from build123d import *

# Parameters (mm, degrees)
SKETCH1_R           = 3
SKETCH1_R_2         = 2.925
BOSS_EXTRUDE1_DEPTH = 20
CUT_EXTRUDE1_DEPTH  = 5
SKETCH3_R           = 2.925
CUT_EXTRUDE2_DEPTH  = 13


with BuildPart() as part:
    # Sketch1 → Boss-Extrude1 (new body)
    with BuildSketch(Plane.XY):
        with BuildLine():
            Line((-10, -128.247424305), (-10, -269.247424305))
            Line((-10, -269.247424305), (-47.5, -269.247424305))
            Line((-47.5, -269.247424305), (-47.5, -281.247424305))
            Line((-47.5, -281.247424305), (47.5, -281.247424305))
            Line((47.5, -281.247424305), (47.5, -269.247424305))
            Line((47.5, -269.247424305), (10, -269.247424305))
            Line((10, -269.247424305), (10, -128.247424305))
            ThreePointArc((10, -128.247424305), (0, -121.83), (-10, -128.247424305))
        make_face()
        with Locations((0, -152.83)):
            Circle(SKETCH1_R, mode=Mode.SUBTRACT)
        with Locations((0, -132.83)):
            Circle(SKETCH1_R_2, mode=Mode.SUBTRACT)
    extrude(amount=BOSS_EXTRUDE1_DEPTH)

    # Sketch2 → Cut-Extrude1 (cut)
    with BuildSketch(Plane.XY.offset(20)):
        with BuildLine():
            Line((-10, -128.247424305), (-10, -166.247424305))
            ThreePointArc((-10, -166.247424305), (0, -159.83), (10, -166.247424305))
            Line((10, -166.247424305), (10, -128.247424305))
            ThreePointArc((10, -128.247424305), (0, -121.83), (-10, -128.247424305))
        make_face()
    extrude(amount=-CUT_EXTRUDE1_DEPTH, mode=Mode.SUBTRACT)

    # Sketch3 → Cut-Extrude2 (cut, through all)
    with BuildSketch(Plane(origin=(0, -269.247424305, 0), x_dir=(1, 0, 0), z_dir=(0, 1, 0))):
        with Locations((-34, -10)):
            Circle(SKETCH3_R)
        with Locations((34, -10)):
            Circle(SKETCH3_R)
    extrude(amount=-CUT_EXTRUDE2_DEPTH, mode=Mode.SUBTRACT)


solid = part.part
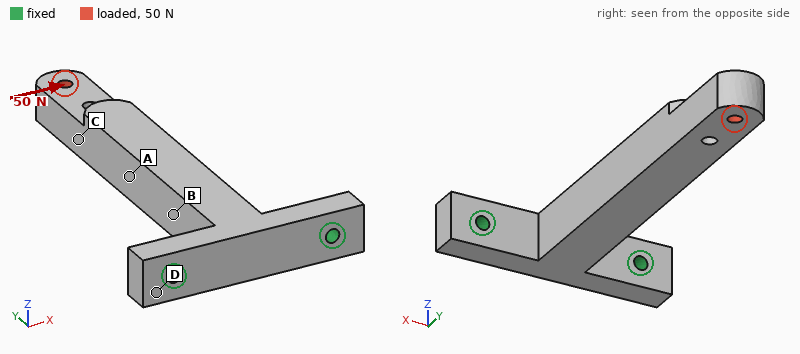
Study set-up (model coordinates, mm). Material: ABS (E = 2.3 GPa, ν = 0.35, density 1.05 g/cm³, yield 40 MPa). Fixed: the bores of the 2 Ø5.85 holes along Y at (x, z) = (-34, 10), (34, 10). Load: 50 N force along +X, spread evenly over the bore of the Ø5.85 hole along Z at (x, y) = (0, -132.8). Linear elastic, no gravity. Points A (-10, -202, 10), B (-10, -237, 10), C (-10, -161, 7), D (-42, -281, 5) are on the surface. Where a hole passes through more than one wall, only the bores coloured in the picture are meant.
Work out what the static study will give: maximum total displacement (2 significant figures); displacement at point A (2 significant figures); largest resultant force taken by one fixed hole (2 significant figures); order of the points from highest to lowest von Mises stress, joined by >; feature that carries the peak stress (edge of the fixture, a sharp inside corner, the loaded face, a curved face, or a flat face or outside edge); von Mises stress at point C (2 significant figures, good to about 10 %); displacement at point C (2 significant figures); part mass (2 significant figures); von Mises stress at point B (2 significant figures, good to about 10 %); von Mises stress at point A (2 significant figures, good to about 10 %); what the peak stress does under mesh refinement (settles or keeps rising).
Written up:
2.1 mm
0.69 mm
150 N
B > A > C > D
edge of the fixture
1.4 MPa
1.4 mm
80 g
3.9 MPa
2.6 MPa
keeps rising
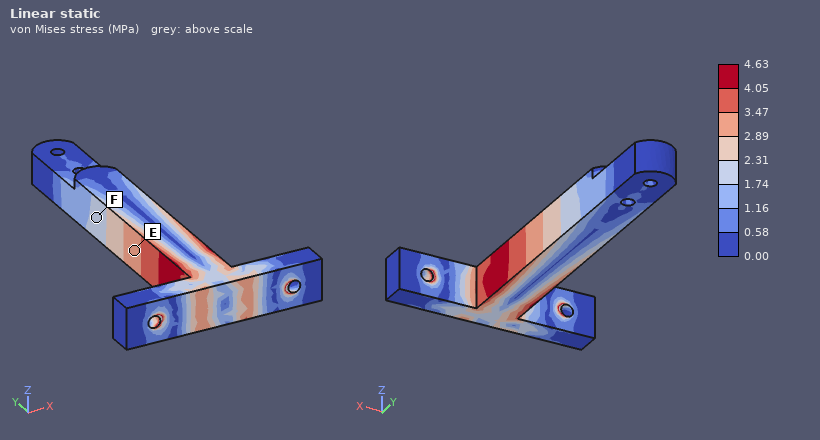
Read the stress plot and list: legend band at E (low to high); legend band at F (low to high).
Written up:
2.89 to 3.47 MPa
1.74 to 2.31 MPa
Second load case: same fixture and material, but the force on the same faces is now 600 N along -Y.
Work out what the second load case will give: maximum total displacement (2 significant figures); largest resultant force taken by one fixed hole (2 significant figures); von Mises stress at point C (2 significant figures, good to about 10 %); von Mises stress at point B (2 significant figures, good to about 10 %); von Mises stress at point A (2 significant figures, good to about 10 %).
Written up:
1.0 mm
310 N
2.4 MPa
1.5 MPa
1.5 MPa
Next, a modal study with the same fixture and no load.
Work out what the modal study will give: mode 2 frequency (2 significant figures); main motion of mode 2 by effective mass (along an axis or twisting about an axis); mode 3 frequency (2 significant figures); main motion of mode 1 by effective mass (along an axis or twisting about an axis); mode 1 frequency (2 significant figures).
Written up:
210 Hz
along X
960 Hz
along Z
140 Hz
